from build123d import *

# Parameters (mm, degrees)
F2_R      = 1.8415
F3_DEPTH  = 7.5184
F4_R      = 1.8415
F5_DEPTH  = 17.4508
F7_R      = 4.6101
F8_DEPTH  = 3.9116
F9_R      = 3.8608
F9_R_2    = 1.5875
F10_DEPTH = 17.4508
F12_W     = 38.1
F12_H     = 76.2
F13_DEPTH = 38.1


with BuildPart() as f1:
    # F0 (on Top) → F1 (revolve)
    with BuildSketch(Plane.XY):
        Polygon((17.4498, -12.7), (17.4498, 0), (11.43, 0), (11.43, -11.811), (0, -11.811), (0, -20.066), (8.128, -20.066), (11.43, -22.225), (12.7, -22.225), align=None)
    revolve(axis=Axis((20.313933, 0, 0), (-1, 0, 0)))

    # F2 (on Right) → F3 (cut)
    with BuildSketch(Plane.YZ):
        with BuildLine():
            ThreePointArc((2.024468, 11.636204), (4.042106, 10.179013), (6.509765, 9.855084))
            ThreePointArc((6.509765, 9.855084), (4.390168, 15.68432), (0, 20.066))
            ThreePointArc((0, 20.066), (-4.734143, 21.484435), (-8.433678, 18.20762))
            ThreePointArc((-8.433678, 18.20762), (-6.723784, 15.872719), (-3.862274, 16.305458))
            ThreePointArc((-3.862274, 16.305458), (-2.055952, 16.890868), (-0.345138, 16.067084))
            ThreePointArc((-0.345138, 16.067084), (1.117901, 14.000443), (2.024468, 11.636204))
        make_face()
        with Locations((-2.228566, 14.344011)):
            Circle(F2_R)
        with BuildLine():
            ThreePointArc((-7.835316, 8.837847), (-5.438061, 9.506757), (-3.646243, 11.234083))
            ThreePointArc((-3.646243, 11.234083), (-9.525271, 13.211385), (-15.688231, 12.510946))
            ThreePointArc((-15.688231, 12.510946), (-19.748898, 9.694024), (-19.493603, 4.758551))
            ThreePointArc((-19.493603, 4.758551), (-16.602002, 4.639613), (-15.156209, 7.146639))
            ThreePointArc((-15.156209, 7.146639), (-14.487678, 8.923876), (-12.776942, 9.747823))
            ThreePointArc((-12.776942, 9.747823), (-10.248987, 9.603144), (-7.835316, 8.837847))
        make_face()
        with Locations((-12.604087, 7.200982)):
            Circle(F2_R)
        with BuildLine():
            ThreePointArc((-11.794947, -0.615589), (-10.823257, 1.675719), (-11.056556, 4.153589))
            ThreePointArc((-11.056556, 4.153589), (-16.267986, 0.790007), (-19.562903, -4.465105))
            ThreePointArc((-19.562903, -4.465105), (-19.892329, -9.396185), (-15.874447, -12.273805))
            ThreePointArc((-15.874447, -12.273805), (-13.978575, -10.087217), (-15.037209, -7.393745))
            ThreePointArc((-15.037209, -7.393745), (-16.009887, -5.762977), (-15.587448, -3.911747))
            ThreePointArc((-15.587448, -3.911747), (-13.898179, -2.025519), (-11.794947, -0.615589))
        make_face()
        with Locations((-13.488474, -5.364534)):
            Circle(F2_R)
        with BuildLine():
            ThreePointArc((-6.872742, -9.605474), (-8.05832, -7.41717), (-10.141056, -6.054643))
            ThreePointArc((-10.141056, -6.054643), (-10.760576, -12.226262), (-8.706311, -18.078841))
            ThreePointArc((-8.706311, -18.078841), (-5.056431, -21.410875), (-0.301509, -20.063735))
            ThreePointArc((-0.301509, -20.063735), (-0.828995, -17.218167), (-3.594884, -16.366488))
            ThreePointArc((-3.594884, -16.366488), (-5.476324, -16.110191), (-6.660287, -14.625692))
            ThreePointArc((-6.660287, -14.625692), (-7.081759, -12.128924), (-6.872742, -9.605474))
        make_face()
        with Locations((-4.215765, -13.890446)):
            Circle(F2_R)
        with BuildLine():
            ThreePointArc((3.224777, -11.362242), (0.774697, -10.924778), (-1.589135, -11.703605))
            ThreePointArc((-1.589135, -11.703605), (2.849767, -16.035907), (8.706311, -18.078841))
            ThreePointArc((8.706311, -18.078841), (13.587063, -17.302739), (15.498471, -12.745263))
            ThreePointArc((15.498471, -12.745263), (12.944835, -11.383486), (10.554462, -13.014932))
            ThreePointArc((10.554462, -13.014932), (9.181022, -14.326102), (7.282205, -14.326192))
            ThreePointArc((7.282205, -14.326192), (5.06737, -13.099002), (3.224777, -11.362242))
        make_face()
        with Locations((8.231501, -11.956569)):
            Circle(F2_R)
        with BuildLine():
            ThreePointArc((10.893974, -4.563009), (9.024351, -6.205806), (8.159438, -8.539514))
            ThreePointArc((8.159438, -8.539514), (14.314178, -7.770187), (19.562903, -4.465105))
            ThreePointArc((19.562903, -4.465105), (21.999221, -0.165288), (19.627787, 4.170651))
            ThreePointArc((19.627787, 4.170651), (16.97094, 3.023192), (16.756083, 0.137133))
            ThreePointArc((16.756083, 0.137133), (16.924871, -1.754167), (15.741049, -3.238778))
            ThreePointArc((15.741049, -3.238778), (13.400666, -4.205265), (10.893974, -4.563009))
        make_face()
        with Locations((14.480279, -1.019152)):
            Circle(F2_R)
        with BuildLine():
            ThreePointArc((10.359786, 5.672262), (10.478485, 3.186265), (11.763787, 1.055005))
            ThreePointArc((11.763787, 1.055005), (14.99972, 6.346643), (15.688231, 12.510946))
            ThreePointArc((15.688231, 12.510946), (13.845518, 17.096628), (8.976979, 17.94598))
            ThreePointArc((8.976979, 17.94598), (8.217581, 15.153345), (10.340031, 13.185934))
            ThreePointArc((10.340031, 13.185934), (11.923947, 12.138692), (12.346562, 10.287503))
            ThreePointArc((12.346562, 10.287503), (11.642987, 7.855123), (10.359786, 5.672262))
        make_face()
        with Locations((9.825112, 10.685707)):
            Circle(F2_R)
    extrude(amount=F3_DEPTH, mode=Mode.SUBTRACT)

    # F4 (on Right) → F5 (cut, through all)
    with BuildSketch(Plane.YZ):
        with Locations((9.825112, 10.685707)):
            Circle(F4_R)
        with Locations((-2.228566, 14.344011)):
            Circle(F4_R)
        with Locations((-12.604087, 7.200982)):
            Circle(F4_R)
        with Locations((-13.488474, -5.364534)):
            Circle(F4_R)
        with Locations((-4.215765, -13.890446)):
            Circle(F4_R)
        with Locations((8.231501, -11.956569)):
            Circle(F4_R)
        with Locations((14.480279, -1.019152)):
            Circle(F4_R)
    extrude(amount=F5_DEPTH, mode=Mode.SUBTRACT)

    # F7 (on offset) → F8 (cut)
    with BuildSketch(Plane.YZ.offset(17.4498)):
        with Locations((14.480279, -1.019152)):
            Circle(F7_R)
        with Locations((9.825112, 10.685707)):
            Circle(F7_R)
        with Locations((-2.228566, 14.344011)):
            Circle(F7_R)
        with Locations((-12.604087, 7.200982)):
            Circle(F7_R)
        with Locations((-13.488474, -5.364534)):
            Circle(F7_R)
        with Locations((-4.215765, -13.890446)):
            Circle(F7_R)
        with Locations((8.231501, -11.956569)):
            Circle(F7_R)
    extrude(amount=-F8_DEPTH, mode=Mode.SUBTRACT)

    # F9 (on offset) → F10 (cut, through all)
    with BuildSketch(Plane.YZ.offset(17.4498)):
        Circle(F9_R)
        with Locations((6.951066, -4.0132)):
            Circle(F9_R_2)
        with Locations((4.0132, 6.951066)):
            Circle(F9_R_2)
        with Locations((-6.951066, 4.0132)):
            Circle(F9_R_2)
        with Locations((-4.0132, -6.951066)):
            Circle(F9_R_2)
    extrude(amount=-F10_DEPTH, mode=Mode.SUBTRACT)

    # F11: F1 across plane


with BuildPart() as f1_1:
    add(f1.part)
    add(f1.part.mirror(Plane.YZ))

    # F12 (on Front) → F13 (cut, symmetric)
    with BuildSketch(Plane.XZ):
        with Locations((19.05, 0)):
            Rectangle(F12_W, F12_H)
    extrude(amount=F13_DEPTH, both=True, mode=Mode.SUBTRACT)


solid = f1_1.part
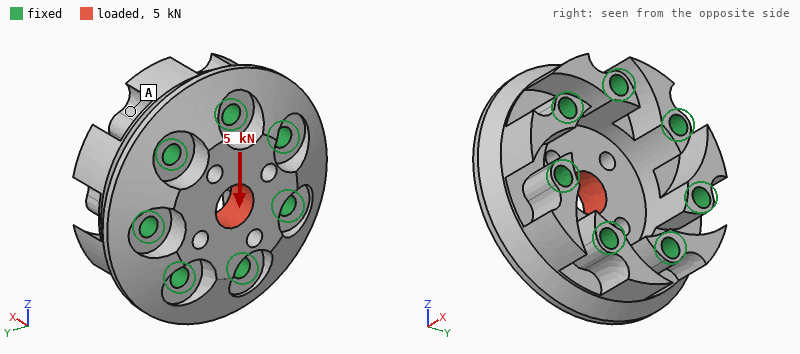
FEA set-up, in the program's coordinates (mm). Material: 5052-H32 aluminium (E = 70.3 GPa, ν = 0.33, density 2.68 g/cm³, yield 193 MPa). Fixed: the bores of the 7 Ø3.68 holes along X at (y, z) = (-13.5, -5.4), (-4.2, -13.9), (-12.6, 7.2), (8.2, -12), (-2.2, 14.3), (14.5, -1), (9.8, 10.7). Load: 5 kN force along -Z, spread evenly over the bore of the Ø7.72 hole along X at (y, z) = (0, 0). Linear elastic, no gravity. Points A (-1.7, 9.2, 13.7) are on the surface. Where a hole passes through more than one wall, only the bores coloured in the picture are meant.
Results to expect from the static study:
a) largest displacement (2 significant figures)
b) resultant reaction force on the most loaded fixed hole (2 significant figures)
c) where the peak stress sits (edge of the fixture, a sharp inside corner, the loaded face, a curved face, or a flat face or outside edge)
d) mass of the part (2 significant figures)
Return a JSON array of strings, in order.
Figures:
["8.5 µm", "1.1 kN", "a curved face", "29 g"]
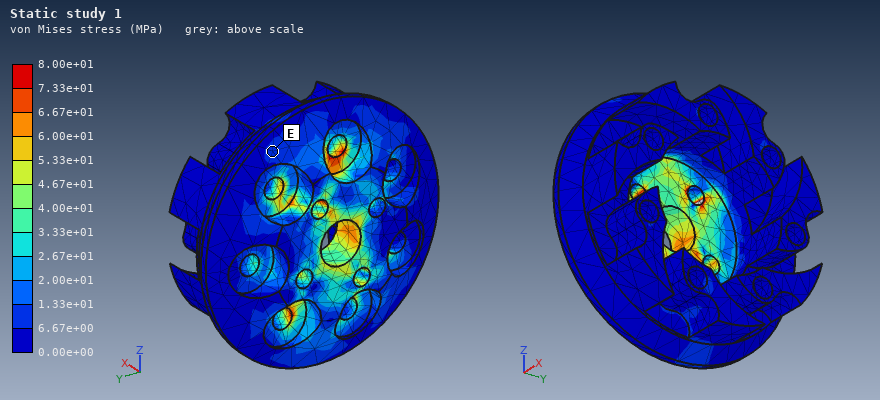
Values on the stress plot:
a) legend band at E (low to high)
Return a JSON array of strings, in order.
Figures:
["6.67e+00 to 1.33e+01 MPa"]
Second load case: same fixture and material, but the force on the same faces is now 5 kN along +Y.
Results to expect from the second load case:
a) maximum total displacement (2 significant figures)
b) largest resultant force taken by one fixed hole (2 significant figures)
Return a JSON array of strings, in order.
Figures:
["8.7 µm", "1.1 kN"]
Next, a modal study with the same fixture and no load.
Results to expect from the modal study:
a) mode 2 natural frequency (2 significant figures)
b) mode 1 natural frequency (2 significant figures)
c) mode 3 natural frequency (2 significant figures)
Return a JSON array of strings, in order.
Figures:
["52 kHz", "48 kHz", "52 kHz"]
